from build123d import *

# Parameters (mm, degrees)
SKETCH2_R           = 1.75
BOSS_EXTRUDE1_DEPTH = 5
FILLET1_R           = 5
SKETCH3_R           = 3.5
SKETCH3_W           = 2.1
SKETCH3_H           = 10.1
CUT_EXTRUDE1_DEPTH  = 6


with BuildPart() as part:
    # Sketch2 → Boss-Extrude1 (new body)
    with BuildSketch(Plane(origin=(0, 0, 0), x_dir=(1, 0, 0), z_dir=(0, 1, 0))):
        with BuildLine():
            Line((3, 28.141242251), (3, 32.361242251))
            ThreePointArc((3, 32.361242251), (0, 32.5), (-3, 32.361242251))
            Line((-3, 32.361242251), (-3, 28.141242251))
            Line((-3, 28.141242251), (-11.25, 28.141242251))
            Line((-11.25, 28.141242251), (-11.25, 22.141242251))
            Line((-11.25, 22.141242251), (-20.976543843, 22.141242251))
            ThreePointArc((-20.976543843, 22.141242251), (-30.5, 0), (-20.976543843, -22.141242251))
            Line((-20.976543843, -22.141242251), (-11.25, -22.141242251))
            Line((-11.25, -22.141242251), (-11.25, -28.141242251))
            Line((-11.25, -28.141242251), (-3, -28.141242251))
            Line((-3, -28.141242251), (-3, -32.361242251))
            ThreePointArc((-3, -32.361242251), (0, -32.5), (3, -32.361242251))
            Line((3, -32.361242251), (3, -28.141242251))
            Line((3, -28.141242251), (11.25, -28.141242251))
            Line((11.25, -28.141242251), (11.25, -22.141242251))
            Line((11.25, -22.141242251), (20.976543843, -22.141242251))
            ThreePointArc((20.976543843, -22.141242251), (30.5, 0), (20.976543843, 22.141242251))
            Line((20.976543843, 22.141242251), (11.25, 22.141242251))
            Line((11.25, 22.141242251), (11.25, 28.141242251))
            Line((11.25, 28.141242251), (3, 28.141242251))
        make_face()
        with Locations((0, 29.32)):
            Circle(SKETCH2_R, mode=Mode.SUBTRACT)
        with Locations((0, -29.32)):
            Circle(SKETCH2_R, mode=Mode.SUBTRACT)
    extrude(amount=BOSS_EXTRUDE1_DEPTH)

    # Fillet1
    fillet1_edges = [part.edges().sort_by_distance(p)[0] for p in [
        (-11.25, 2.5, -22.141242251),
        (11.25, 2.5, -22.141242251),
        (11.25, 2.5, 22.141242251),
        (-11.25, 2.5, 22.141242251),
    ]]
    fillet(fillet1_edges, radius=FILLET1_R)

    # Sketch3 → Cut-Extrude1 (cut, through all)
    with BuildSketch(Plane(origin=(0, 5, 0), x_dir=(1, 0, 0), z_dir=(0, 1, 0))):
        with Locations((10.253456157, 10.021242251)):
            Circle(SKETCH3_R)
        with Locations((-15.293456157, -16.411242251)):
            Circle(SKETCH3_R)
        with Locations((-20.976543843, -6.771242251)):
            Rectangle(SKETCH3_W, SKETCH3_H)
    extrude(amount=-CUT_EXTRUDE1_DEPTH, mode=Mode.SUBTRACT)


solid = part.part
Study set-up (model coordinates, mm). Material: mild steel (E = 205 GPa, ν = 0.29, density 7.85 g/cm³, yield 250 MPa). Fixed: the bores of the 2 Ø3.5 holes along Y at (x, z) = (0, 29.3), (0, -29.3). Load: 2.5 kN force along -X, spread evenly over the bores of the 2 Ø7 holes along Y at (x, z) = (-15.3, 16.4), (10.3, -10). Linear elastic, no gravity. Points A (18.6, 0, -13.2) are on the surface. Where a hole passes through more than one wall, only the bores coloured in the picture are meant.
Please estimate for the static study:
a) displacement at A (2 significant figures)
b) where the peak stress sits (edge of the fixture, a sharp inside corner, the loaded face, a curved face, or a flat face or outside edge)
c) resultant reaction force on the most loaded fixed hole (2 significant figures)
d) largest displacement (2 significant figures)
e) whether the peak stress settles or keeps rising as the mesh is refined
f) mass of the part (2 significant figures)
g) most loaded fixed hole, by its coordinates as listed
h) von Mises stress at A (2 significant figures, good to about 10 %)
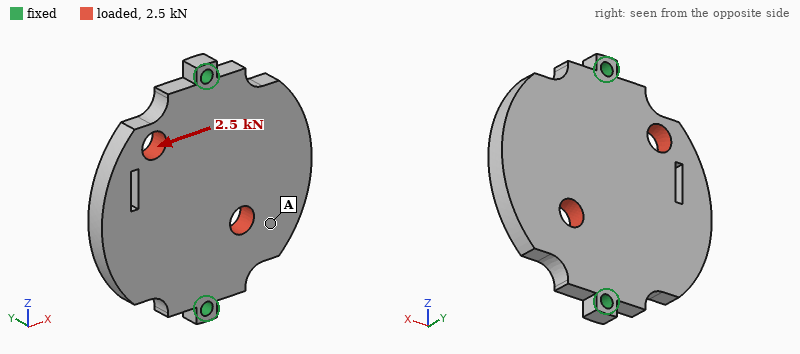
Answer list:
2.9 µm
edge of the fixture
1.4 kN
4.1 µm
keeps rising
100 g
(0, 29.3)
12 MPa
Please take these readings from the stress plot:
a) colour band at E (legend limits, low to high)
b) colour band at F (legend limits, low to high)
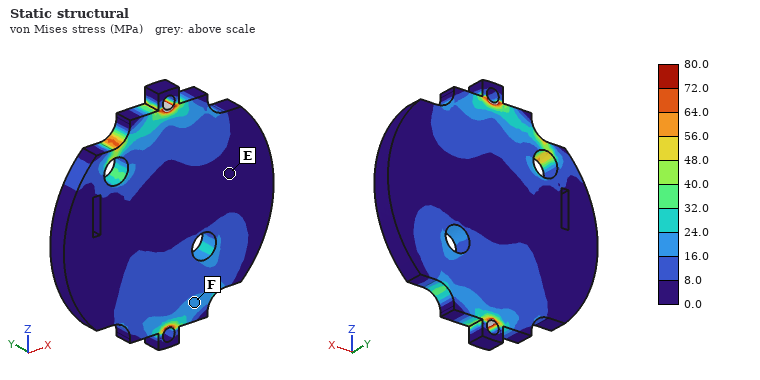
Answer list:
0.0 to 8.0 MPa
16.0 to 24.0 MPa
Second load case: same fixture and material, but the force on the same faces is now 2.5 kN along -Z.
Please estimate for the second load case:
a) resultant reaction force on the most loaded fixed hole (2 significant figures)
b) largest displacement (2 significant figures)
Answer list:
1.3 kN
3.8 µm
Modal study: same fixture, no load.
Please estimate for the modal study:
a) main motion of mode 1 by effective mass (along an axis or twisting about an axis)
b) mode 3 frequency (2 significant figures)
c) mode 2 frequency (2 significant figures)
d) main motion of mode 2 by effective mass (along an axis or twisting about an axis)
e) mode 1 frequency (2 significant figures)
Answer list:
twisting about Z
9100 Hz
3800 Hz
along Y
2500 Hz
